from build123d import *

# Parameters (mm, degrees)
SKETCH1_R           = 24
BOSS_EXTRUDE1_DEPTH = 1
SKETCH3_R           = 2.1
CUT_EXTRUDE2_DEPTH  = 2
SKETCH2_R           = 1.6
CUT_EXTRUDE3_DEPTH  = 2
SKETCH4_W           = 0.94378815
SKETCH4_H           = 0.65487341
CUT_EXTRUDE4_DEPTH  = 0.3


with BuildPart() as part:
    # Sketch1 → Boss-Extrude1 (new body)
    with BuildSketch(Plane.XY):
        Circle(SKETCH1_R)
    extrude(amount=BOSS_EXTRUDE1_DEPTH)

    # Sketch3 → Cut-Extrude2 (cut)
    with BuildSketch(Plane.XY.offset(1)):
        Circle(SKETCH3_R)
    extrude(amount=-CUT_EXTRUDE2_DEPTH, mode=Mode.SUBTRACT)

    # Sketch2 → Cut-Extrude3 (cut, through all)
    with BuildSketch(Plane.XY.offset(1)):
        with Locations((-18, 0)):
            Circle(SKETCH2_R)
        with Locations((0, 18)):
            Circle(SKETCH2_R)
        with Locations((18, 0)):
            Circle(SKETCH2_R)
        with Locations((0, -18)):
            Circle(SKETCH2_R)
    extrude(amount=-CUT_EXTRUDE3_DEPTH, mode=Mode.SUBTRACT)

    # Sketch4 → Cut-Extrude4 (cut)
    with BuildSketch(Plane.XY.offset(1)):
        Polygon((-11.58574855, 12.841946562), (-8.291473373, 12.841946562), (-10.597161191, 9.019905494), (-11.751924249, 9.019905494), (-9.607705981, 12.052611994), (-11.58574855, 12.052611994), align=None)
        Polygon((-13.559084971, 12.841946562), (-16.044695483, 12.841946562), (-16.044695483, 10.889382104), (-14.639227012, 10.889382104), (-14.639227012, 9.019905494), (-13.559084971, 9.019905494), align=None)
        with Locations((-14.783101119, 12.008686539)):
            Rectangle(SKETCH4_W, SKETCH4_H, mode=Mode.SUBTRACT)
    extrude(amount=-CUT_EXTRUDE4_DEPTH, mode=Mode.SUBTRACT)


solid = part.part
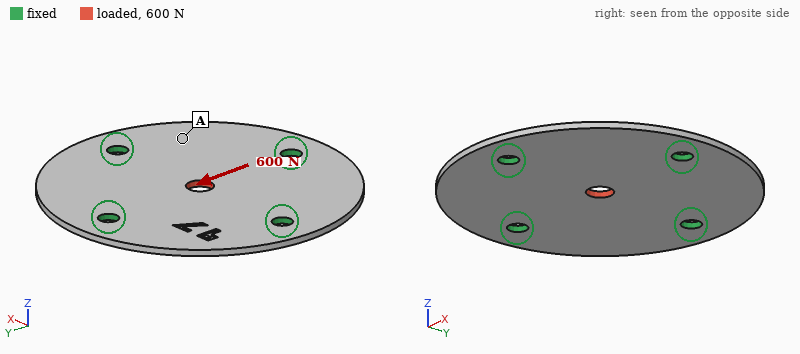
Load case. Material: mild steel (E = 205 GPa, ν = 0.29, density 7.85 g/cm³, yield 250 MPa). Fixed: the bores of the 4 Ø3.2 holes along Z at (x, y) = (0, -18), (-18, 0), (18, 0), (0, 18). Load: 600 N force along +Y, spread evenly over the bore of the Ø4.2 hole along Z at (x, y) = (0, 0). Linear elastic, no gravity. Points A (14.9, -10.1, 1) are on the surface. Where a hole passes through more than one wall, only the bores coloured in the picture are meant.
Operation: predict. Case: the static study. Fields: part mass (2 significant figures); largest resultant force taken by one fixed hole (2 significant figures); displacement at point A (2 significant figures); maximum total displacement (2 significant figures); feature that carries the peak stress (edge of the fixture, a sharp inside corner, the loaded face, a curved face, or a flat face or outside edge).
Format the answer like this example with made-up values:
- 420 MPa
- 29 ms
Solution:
- 14 g
- 200 N
- 0.48 µm
- 2.0 µm
- the loaded face
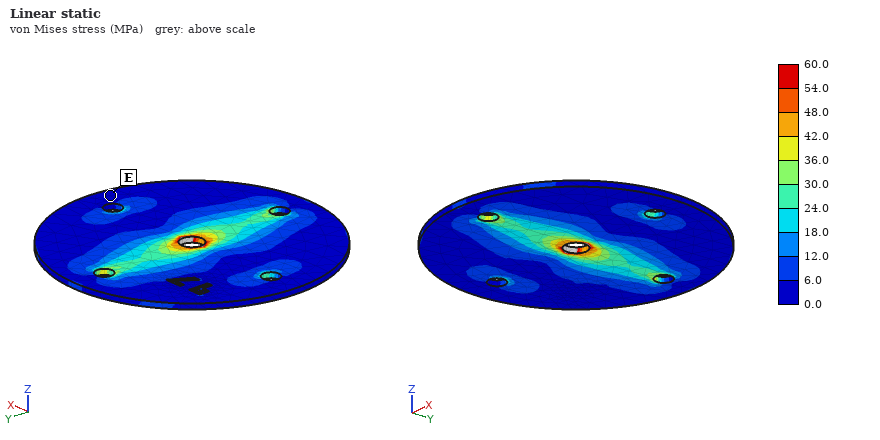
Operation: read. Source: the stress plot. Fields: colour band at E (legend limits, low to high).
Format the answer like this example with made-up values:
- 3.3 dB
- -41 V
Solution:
- 0.0 to 6.0 MPa
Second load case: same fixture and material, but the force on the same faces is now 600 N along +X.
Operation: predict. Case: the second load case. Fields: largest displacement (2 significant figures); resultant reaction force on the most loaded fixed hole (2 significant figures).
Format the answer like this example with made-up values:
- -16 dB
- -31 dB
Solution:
- 2.0 µm
- 200 N
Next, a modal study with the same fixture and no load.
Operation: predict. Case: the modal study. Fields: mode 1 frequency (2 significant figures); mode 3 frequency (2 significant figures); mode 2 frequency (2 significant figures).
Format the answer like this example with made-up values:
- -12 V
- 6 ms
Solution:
- 6000 Hz
- 6200 Hz
- 6200 Hz
